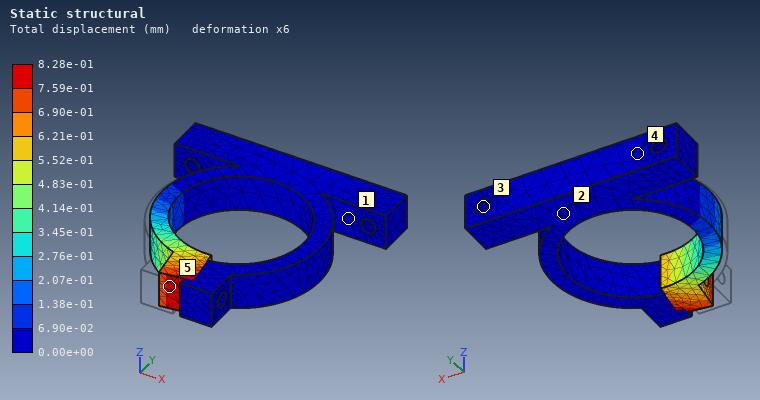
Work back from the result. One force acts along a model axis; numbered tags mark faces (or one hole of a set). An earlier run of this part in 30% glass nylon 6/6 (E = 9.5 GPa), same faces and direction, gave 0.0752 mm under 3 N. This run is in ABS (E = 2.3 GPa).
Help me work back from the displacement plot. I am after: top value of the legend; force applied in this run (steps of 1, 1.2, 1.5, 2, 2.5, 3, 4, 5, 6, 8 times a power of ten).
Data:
8.28e-01 mm
8 N
